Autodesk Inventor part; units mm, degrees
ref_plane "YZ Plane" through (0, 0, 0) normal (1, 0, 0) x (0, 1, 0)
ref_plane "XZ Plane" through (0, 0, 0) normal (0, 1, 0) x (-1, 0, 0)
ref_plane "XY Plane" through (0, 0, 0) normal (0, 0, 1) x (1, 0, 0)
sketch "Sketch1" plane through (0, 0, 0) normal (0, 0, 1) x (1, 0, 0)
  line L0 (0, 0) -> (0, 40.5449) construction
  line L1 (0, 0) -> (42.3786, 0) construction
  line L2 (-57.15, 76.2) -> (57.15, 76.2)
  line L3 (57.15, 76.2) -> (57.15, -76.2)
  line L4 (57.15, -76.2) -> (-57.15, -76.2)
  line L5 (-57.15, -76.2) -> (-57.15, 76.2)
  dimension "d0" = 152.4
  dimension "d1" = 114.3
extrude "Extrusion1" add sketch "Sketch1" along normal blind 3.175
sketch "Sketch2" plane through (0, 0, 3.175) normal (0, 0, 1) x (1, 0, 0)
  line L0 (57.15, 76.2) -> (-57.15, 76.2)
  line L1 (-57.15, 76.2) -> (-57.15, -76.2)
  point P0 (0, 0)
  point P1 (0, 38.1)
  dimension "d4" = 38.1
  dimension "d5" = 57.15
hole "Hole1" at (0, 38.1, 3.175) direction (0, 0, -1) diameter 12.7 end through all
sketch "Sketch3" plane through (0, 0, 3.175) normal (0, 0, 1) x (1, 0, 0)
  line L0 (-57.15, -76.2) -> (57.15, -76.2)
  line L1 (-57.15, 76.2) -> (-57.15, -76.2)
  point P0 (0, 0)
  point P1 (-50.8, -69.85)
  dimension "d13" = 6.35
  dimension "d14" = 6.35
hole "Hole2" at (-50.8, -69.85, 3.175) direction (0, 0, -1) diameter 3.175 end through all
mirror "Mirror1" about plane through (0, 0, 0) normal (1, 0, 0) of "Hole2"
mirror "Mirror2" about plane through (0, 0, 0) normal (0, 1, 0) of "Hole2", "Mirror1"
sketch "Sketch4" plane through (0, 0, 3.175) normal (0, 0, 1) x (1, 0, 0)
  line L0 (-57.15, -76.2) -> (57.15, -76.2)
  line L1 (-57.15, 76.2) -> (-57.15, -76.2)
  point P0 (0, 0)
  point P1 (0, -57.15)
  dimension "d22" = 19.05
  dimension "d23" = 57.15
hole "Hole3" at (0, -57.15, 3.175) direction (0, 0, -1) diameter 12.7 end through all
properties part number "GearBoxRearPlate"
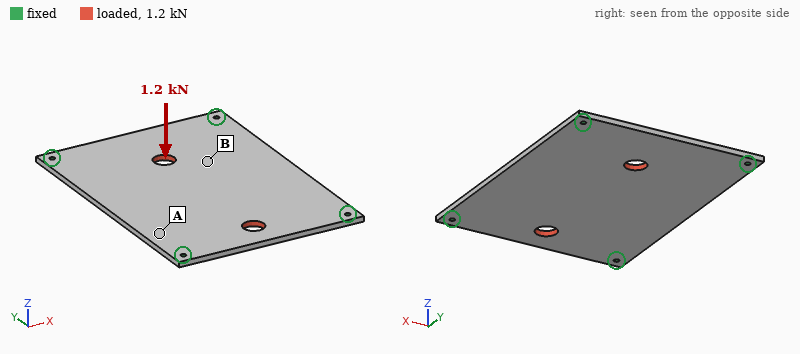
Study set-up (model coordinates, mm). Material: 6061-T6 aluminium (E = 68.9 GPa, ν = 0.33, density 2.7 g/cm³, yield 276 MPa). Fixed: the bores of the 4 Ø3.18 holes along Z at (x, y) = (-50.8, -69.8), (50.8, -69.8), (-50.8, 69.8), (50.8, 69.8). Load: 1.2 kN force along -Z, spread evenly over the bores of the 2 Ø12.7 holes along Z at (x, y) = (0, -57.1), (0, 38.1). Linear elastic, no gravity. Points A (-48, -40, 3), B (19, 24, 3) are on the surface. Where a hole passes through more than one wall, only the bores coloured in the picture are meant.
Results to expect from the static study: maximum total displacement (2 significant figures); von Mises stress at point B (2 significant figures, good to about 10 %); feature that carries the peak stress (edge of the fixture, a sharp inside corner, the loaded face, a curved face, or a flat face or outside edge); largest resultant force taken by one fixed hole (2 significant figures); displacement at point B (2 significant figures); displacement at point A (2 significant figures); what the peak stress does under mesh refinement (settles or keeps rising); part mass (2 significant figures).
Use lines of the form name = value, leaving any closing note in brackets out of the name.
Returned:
maximum total displacement = 0.80 mm
von Mises stress at point B = 49 MPa
feature that carries the peak stress = edge of the fixture
largest resultant force taken by one fixed hole = 340 N
displacement at point B = 0.70 mm
displacement at point A = 0.23 mm
what the peak stress does under mesh refinement = keeps rising
part mass = 150 g
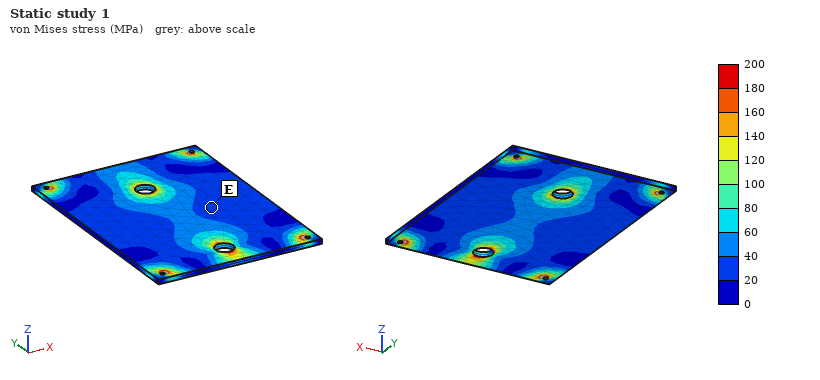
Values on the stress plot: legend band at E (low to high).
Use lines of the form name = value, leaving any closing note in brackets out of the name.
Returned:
legend band at E = 20 to 40 MPa
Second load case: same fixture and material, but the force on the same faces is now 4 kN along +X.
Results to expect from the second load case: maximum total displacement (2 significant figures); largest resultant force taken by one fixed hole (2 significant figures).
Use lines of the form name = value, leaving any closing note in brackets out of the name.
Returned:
maximum total displacement = 15 µm
largest resultant force taken by one fixed hole = 1.2 kN
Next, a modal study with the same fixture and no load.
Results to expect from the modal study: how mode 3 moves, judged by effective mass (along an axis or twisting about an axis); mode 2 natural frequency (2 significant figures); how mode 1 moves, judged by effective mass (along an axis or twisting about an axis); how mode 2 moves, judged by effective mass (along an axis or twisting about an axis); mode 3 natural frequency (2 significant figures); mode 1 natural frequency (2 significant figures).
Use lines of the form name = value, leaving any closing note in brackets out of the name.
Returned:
how mode 3 moves, judged by effective mass = twisting about X
mode 2 natural frequency = 1000 Hz
how mode 1 moves, judged by effective mass = along Z
how mode 2 moves, judged by effective mass = twisting about Y
mode 3 natural frequency = 1400 Hz
mode 1 natural frequency = 610 Hz
